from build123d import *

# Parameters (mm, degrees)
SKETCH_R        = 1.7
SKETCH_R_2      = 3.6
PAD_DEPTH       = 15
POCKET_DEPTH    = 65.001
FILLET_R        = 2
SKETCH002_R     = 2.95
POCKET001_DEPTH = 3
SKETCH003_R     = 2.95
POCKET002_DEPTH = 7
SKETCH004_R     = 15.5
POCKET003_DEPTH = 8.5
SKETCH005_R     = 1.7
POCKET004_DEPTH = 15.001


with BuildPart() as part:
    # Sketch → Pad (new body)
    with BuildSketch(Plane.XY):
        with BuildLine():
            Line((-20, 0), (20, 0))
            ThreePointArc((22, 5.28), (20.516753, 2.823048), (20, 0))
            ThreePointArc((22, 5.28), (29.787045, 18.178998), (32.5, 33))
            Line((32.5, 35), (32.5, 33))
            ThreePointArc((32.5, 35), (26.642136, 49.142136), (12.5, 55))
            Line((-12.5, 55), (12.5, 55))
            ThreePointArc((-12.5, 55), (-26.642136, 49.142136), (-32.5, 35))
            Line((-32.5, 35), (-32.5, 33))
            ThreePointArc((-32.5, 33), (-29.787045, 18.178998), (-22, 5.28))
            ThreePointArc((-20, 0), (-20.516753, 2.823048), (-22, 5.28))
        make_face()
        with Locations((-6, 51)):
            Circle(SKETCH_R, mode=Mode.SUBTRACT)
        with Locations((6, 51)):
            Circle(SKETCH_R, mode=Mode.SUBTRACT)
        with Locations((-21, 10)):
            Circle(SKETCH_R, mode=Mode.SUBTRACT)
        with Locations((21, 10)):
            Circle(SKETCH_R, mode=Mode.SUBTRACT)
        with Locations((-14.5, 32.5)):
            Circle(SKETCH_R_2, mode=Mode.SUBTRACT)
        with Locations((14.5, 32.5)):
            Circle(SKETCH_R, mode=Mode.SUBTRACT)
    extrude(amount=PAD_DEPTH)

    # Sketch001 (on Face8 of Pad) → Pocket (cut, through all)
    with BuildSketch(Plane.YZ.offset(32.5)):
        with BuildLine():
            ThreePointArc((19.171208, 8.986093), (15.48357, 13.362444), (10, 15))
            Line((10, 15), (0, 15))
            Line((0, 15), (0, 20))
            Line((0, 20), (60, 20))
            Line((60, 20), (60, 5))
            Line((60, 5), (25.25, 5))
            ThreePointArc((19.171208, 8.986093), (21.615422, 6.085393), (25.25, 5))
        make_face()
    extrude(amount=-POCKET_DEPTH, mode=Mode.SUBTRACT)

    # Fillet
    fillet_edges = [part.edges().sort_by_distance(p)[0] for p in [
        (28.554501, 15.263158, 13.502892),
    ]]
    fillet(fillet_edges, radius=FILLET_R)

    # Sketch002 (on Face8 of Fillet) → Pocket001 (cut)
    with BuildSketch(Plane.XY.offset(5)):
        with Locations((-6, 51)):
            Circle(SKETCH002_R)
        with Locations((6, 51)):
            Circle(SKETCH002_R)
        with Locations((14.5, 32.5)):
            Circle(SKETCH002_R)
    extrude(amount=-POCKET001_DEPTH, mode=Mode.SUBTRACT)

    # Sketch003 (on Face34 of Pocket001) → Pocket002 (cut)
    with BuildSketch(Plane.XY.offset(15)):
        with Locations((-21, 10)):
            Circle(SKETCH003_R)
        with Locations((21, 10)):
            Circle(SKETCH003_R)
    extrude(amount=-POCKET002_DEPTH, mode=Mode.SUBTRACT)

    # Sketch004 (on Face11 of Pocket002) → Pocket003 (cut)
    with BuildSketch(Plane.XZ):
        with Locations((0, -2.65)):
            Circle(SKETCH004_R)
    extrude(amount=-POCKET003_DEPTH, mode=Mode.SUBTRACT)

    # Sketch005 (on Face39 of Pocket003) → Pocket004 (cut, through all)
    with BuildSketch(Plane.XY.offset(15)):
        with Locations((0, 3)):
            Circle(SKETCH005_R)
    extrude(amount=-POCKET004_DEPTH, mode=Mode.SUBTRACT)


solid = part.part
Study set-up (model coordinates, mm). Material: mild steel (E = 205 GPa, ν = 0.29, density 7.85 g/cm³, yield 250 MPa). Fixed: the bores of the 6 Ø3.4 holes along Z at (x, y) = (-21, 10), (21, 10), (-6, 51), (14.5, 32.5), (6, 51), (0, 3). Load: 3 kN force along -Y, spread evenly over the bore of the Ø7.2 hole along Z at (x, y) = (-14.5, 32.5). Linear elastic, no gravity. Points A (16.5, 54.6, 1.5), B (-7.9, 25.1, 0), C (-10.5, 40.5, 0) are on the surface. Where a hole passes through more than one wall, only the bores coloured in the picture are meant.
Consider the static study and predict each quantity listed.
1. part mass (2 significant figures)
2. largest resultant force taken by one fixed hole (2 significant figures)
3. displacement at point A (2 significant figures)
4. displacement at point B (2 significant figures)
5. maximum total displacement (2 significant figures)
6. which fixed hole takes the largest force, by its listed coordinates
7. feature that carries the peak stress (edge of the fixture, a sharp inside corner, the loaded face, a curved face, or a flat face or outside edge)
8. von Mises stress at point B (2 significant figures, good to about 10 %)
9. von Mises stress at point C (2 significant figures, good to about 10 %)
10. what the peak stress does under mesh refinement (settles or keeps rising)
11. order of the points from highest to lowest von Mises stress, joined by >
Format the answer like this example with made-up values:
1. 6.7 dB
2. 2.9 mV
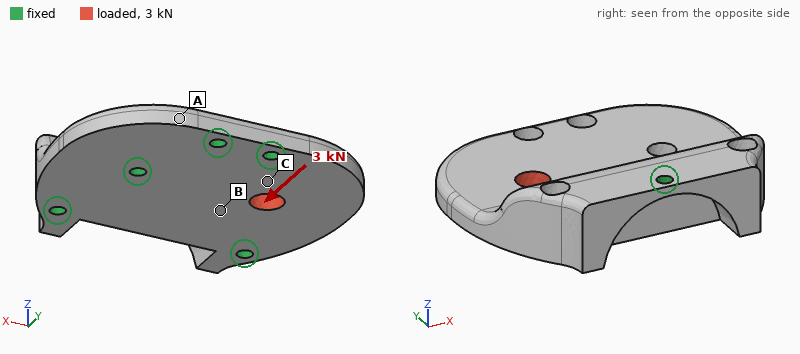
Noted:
1. 160 g
2. 1.6 kN
3. 0.66 µm
4. 2.0 µm
5. 3.4 µm
6. (-21, 10)
7. edge of the fixture
8. 13 MPa
9. 23 MPa
10. keeps rising
11. C > B > A
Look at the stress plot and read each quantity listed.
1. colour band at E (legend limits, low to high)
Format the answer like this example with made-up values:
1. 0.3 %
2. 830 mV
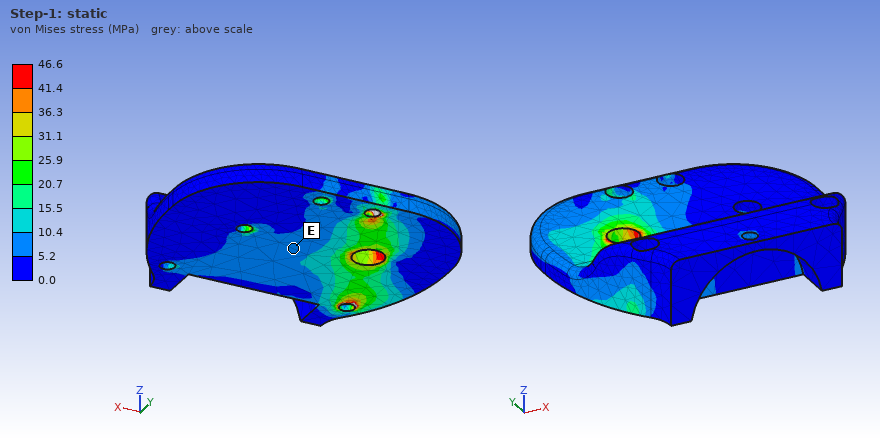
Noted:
1. 5.2 to 10.4 MPa
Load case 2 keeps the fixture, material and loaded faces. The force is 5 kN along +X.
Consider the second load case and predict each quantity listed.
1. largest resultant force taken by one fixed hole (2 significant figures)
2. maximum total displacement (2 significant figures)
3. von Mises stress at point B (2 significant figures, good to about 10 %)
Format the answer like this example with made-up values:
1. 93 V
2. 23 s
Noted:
1. 1.2 kN
2. 4.8 µm
3. 29 MPa
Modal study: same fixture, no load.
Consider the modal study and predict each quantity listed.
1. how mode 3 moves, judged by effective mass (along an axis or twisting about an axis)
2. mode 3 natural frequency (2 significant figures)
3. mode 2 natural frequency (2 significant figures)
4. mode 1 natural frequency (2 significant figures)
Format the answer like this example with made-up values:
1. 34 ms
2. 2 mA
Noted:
1. along Z
2. 17 kHz
3. 11 kHz
4. 8700 Hz
